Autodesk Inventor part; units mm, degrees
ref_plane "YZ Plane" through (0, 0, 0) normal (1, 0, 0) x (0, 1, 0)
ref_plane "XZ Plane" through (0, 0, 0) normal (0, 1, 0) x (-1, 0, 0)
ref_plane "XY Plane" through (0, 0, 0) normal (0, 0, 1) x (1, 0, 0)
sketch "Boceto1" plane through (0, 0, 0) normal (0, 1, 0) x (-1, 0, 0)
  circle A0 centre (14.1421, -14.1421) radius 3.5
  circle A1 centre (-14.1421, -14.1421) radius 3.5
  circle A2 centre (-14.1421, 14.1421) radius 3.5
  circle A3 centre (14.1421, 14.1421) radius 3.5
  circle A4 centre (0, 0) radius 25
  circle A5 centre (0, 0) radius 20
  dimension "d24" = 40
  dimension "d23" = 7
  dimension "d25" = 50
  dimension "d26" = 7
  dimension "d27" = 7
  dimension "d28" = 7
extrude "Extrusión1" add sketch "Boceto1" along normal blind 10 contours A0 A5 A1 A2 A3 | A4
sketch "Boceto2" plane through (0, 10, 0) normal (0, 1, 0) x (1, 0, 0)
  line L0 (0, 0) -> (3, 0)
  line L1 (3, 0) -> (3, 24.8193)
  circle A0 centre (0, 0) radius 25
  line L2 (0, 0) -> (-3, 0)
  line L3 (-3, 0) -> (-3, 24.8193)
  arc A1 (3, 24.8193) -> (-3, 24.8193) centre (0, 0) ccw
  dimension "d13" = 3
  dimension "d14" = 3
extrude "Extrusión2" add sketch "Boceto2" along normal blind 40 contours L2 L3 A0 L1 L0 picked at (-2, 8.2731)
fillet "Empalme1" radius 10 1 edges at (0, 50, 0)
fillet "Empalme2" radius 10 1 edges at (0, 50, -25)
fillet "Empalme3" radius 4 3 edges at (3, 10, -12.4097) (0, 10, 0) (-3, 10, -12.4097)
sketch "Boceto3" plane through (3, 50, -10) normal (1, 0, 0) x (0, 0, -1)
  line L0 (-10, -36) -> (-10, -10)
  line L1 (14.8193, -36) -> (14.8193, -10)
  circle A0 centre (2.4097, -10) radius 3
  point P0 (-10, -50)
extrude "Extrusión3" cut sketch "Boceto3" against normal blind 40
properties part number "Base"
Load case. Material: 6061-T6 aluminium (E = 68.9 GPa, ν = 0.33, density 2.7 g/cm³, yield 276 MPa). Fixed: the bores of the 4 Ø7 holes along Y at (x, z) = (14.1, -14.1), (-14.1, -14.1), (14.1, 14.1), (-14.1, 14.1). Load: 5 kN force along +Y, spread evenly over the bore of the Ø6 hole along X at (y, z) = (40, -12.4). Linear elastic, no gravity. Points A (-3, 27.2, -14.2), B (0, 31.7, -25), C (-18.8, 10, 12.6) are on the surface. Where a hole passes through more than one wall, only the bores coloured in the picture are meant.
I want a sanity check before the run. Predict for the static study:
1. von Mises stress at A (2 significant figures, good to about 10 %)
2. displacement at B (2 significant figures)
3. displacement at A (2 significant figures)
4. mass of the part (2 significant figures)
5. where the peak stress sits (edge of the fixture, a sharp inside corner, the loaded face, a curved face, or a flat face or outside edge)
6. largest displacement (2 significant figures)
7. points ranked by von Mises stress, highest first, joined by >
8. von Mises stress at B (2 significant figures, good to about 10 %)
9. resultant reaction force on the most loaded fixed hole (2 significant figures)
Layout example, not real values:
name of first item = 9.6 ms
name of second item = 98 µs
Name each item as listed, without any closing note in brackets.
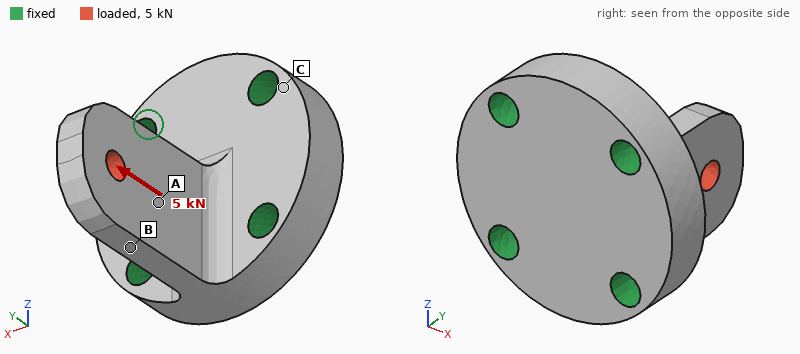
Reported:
von Mises stress at A = 40 MPa
displacement at B = 21 µm
displacement at A = 16 µm
mass of the part = 64 g
where the peak stress sits = the loaded face
largest displacement = 29 µm
points ranked by von Mises stress, highest first, joined by > = A > B > C
von Mises stress at B = 22 MPa
resultant reaction force on the most loaded fixed hole = 2.2 kN
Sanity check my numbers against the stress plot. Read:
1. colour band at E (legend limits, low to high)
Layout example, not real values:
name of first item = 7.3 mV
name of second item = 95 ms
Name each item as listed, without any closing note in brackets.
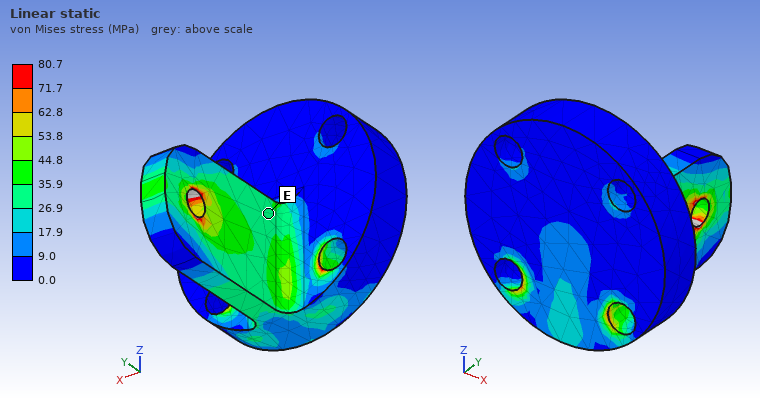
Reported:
colour band at E = 26.9 to 35.9 MPa
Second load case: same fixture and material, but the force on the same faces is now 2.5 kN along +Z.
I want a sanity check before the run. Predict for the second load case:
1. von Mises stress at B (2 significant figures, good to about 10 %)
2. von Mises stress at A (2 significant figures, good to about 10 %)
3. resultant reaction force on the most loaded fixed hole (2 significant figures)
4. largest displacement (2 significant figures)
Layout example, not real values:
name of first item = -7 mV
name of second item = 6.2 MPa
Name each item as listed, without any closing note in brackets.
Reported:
von Mises stress at B = 36 MPa
von Mises stress at A = 44 MPa
resultant reaction force on the most loaded fixed hole = 1.4 kN
largest displacement = 0.14 mm
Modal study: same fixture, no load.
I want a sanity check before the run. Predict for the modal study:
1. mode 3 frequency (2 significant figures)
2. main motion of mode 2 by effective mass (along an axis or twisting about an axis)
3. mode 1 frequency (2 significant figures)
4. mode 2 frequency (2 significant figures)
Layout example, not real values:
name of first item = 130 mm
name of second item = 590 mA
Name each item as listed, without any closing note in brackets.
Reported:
mode 3 frequency = 11 kHz
main motion of mode 2 by effective mass = along Z
mode 1 frequency = 3500 Hz
mode 2 frequency = 8400 Hz
